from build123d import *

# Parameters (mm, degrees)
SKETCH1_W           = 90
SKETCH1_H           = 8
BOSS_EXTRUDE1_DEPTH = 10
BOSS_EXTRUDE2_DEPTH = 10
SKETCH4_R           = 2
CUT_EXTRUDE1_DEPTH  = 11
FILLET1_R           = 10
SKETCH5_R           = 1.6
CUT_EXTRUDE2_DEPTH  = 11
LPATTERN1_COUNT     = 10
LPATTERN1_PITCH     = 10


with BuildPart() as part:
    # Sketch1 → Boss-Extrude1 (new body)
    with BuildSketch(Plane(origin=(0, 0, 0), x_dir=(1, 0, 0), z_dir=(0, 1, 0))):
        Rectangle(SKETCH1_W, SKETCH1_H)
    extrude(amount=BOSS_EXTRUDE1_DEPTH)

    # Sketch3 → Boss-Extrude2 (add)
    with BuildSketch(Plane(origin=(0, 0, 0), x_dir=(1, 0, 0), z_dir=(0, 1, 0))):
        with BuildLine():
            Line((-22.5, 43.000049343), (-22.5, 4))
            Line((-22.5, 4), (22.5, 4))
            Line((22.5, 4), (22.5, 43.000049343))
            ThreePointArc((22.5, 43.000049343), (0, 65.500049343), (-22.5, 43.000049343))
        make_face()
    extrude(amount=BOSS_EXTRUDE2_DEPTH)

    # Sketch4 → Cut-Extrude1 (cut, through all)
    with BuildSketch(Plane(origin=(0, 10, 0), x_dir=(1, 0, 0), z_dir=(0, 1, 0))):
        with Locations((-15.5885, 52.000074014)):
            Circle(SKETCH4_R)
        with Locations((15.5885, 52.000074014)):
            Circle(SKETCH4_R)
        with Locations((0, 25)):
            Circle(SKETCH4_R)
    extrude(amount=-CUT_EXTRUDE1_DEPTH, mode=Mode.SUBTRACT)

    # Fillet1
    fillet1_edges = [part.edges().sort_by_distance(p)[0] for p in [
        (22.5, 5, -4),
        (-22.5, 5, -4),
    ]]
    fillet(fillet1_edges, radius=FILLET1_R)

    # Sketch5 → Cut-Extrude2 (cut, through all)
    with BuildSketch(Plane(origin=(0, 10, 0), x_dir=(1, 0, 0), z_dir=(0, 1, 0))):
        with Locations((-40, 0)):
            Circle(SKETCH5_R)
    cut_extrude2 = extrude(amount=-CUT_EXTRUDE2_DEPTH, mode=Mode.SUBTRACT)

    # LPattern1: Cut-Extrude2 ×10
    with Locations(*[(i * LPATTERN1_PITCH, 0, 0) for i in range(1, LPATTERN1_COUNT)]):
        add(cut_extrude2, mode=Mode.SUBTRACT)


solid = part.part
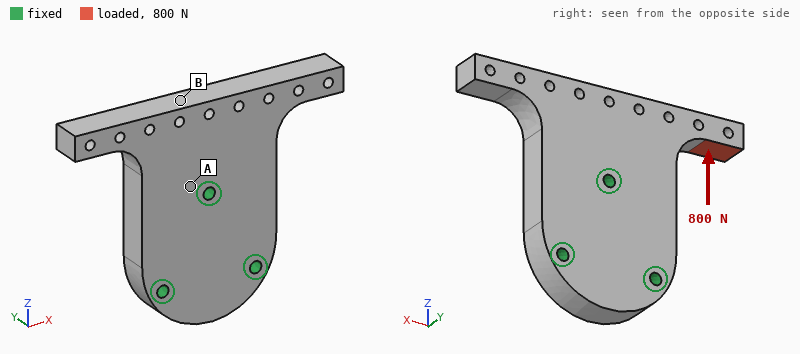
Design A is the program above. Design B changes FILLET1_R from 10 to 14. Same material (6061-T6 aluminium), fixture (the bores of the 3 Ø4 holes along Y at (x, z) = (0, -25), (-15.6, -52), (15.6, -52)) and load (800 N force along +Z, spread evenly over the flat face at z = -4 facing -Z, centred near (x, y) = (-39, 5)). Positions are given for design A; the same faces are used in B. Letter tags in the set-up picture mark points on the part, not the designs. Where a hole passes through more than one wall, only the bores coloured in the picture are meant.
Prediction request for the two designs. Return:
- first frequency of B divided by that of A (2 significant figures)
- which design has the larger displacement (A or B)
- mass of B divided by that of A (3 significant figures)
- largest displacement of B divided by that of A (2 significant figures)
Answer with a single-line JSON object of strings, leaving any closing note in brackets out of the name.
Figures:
{"first frequency of B divided by that of A": "1.0", "which design has the larger displacement": "A", "mass of B divided by that of A": "1.01", "largest displacement of B divided by that of A": "0.89"}
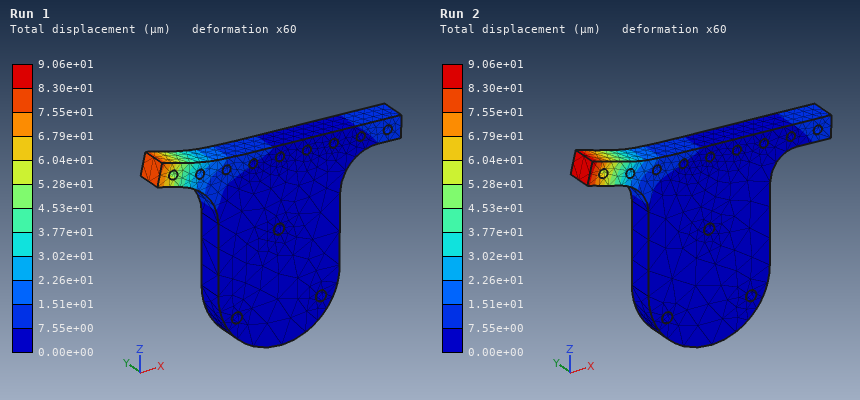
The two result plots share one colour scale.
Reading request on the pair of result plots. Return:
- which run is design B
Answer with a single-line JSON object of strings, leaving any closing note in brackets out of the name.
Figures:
{"which run is design B": "Run 1"}
